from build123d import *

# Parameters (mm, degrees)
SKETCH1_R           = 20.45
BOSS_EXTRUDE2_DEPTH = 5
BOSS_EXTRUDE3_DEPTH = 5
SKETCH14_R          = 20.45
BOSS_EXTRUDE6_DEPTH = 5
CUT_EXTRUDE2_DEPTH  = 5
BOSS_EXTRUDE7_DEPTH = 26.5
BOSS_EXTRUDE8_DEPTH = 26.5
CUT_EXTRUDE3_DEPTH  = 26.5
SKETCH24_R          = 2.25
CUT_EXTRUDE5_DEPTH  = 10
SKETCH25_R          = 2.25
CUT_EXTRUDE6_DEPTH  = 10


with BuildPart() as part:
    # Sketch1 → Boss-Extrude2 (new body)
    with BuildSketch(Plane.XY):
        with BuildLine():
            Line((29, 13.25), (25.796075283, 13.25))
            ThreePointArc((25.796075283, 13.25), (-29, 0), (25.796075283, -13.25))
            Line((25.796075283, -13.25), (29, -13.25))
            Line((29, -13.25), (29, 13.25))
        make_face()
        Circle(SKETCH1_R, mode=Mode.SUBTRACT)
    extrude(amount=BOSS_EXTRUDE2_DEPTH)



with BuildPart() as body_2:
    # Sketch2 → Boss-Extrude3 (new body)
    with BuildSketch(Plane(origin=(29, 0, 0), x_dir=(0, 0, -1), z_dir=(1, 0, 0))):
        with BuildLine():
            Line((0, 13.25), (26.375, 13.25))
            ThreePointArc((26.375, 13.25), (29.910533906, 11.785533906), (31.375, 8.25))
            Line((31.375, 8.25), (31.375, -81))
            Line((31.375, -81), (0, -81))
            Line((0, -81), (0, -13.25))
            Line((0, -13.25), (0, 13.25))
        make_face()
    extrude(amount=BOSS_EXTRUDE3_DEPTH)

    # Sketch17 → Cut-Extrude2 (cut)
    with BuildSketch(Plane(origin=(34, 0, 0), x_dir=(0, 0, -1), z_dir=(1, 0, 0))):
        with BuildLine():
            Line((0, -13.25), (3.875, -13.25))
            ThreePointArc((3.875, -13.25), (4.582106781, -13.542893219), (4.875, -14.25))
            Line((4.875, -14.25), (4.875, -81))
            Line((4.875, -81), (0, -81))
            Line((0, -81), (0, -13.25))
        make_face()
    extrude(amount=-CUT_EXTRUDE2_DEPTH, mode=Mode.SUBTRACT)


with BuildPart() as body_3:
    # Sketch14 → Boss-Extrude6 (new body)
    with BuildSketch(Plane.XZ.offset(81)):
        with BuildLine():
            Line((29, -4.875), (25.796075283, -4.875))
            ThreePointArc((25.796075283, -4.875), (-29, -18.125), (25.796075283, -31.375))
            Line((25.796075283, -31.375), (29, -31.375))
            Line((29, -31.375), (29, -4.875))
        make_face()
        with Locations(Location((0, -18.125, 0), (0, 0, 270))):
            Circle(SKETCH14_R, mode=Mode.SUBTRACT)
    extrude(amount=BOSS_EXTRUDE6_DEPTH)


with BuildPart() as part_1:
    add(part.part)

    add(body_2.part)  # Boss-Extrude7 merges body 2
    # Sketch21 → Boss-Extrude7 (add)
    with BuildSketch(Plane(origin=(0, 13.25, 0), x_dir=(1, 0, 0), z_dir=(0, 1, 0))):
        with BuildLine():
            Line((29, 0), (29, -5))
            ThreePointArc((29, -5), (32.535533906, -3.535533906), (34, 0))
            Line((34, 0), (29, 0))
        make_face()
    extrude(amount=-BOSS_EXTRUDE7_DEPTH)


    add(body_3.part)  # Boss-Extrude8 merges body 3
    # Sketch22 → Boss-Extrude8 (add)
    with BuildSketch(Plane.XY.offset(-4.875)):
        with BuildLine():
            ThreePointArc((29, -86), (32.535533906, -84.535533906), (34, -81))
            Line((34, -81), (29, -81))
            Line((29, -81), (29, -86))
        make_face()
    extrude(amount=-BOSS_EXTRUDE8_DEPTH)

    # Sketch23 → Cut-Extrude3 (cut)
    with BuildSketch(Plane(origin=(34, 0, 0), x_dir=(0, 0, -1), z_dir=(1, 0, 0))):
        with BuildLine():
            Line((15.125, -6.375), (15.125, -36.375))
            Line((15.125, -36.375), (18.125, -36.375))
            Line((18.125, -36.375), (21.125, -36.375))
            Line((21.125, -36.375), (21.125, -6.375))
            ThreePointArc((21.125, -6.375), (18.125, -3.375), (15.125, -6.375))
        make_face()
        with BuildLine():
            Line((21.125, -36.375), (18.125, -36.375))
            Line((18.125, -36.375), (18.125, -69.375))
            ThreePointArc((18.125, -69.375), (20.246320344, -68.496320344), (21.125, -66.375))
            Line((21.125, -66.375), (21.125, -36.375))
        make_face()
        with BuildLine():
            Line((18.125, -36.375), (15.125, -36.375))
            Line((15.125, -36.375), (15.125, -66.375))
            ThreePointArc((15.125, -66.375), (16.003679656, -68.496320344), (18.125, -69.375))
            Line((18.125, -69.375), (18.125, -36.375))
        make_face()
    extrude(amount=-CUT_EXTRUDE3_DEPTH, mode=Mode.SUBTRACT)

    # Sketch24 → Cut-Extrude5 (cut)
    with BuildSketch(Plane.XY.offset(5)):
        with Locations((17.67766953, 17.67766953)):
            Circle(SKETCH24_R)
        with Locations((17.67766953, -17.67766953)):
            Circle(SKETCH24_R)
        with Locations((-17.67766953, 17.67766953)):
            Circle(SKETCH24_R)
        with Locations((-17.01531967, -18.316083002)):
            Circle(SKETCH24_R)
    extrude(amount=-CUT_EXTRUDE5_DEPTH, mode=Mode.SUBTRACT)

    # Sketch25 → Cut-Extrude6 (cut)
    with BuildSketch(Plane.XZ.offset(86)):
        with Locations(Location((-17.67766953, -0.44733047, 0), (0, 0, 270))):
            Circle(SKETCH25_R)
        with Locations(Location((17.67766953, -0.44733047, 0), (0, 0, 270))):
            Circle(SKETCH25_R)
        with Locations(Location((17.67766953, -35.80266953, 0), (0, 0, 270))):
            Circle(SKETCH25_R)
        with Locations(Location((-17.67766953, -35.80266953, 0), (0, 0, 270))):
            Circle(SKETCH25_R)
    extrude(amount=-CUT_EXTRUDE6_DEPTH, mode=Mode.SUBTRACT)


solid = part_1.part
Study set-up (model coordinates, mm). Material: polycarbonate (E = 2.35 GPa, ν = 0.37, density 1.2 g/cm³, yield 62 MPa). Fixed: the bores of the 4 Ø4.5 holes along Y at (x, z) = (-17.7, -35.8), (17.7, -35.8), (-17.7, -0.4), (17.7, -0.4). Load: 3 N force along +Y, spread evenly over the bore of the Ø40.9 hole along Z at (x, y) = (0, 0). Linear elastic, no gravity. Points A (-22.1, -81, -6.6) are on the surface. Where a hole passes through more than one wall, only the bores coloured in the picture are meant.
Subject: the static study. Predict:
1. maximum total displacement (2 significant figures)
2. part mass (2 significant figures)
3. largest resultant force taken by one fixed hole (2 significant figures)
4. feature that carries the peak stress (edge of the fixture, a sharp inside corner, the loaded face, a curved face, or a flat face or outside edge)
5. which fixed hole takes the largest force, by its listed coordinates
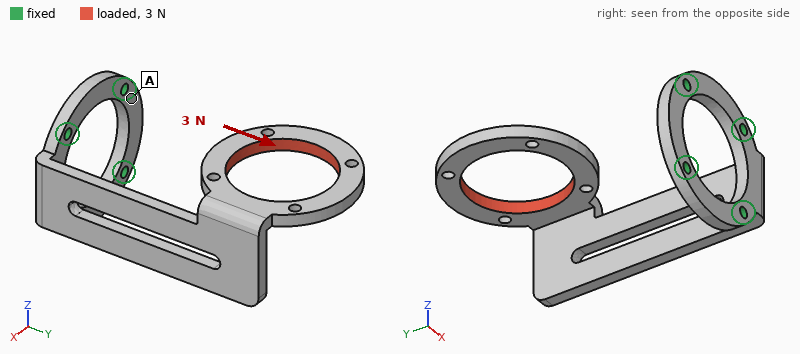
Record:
1.5 mm
30 g
3.8 N
a curved face
(17.7, -0.4)
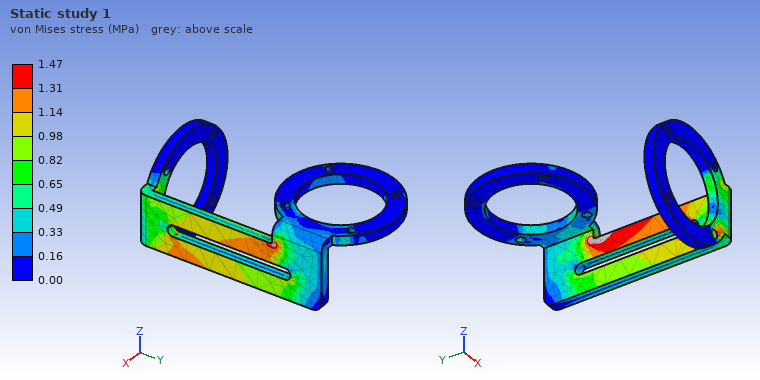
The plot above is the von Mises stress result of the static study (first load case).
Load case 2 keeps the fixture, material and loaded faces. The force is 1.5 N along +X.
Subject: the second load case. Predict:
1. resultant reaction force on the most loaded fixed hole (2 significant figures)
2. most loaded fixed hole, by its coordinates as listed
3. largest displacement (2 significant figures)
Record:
2.3 N
(17.7, -0.4)
1.4 mm
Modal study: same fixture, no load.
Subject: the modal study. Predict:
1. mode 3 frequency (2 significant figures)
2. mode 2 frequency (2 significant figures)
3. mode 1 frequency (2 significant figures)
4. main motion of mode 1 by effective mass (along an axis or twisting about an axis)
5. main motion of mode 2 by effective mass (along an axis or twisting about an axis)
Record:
190 Hz
95 Hz
50 Hz
along X
along Z
